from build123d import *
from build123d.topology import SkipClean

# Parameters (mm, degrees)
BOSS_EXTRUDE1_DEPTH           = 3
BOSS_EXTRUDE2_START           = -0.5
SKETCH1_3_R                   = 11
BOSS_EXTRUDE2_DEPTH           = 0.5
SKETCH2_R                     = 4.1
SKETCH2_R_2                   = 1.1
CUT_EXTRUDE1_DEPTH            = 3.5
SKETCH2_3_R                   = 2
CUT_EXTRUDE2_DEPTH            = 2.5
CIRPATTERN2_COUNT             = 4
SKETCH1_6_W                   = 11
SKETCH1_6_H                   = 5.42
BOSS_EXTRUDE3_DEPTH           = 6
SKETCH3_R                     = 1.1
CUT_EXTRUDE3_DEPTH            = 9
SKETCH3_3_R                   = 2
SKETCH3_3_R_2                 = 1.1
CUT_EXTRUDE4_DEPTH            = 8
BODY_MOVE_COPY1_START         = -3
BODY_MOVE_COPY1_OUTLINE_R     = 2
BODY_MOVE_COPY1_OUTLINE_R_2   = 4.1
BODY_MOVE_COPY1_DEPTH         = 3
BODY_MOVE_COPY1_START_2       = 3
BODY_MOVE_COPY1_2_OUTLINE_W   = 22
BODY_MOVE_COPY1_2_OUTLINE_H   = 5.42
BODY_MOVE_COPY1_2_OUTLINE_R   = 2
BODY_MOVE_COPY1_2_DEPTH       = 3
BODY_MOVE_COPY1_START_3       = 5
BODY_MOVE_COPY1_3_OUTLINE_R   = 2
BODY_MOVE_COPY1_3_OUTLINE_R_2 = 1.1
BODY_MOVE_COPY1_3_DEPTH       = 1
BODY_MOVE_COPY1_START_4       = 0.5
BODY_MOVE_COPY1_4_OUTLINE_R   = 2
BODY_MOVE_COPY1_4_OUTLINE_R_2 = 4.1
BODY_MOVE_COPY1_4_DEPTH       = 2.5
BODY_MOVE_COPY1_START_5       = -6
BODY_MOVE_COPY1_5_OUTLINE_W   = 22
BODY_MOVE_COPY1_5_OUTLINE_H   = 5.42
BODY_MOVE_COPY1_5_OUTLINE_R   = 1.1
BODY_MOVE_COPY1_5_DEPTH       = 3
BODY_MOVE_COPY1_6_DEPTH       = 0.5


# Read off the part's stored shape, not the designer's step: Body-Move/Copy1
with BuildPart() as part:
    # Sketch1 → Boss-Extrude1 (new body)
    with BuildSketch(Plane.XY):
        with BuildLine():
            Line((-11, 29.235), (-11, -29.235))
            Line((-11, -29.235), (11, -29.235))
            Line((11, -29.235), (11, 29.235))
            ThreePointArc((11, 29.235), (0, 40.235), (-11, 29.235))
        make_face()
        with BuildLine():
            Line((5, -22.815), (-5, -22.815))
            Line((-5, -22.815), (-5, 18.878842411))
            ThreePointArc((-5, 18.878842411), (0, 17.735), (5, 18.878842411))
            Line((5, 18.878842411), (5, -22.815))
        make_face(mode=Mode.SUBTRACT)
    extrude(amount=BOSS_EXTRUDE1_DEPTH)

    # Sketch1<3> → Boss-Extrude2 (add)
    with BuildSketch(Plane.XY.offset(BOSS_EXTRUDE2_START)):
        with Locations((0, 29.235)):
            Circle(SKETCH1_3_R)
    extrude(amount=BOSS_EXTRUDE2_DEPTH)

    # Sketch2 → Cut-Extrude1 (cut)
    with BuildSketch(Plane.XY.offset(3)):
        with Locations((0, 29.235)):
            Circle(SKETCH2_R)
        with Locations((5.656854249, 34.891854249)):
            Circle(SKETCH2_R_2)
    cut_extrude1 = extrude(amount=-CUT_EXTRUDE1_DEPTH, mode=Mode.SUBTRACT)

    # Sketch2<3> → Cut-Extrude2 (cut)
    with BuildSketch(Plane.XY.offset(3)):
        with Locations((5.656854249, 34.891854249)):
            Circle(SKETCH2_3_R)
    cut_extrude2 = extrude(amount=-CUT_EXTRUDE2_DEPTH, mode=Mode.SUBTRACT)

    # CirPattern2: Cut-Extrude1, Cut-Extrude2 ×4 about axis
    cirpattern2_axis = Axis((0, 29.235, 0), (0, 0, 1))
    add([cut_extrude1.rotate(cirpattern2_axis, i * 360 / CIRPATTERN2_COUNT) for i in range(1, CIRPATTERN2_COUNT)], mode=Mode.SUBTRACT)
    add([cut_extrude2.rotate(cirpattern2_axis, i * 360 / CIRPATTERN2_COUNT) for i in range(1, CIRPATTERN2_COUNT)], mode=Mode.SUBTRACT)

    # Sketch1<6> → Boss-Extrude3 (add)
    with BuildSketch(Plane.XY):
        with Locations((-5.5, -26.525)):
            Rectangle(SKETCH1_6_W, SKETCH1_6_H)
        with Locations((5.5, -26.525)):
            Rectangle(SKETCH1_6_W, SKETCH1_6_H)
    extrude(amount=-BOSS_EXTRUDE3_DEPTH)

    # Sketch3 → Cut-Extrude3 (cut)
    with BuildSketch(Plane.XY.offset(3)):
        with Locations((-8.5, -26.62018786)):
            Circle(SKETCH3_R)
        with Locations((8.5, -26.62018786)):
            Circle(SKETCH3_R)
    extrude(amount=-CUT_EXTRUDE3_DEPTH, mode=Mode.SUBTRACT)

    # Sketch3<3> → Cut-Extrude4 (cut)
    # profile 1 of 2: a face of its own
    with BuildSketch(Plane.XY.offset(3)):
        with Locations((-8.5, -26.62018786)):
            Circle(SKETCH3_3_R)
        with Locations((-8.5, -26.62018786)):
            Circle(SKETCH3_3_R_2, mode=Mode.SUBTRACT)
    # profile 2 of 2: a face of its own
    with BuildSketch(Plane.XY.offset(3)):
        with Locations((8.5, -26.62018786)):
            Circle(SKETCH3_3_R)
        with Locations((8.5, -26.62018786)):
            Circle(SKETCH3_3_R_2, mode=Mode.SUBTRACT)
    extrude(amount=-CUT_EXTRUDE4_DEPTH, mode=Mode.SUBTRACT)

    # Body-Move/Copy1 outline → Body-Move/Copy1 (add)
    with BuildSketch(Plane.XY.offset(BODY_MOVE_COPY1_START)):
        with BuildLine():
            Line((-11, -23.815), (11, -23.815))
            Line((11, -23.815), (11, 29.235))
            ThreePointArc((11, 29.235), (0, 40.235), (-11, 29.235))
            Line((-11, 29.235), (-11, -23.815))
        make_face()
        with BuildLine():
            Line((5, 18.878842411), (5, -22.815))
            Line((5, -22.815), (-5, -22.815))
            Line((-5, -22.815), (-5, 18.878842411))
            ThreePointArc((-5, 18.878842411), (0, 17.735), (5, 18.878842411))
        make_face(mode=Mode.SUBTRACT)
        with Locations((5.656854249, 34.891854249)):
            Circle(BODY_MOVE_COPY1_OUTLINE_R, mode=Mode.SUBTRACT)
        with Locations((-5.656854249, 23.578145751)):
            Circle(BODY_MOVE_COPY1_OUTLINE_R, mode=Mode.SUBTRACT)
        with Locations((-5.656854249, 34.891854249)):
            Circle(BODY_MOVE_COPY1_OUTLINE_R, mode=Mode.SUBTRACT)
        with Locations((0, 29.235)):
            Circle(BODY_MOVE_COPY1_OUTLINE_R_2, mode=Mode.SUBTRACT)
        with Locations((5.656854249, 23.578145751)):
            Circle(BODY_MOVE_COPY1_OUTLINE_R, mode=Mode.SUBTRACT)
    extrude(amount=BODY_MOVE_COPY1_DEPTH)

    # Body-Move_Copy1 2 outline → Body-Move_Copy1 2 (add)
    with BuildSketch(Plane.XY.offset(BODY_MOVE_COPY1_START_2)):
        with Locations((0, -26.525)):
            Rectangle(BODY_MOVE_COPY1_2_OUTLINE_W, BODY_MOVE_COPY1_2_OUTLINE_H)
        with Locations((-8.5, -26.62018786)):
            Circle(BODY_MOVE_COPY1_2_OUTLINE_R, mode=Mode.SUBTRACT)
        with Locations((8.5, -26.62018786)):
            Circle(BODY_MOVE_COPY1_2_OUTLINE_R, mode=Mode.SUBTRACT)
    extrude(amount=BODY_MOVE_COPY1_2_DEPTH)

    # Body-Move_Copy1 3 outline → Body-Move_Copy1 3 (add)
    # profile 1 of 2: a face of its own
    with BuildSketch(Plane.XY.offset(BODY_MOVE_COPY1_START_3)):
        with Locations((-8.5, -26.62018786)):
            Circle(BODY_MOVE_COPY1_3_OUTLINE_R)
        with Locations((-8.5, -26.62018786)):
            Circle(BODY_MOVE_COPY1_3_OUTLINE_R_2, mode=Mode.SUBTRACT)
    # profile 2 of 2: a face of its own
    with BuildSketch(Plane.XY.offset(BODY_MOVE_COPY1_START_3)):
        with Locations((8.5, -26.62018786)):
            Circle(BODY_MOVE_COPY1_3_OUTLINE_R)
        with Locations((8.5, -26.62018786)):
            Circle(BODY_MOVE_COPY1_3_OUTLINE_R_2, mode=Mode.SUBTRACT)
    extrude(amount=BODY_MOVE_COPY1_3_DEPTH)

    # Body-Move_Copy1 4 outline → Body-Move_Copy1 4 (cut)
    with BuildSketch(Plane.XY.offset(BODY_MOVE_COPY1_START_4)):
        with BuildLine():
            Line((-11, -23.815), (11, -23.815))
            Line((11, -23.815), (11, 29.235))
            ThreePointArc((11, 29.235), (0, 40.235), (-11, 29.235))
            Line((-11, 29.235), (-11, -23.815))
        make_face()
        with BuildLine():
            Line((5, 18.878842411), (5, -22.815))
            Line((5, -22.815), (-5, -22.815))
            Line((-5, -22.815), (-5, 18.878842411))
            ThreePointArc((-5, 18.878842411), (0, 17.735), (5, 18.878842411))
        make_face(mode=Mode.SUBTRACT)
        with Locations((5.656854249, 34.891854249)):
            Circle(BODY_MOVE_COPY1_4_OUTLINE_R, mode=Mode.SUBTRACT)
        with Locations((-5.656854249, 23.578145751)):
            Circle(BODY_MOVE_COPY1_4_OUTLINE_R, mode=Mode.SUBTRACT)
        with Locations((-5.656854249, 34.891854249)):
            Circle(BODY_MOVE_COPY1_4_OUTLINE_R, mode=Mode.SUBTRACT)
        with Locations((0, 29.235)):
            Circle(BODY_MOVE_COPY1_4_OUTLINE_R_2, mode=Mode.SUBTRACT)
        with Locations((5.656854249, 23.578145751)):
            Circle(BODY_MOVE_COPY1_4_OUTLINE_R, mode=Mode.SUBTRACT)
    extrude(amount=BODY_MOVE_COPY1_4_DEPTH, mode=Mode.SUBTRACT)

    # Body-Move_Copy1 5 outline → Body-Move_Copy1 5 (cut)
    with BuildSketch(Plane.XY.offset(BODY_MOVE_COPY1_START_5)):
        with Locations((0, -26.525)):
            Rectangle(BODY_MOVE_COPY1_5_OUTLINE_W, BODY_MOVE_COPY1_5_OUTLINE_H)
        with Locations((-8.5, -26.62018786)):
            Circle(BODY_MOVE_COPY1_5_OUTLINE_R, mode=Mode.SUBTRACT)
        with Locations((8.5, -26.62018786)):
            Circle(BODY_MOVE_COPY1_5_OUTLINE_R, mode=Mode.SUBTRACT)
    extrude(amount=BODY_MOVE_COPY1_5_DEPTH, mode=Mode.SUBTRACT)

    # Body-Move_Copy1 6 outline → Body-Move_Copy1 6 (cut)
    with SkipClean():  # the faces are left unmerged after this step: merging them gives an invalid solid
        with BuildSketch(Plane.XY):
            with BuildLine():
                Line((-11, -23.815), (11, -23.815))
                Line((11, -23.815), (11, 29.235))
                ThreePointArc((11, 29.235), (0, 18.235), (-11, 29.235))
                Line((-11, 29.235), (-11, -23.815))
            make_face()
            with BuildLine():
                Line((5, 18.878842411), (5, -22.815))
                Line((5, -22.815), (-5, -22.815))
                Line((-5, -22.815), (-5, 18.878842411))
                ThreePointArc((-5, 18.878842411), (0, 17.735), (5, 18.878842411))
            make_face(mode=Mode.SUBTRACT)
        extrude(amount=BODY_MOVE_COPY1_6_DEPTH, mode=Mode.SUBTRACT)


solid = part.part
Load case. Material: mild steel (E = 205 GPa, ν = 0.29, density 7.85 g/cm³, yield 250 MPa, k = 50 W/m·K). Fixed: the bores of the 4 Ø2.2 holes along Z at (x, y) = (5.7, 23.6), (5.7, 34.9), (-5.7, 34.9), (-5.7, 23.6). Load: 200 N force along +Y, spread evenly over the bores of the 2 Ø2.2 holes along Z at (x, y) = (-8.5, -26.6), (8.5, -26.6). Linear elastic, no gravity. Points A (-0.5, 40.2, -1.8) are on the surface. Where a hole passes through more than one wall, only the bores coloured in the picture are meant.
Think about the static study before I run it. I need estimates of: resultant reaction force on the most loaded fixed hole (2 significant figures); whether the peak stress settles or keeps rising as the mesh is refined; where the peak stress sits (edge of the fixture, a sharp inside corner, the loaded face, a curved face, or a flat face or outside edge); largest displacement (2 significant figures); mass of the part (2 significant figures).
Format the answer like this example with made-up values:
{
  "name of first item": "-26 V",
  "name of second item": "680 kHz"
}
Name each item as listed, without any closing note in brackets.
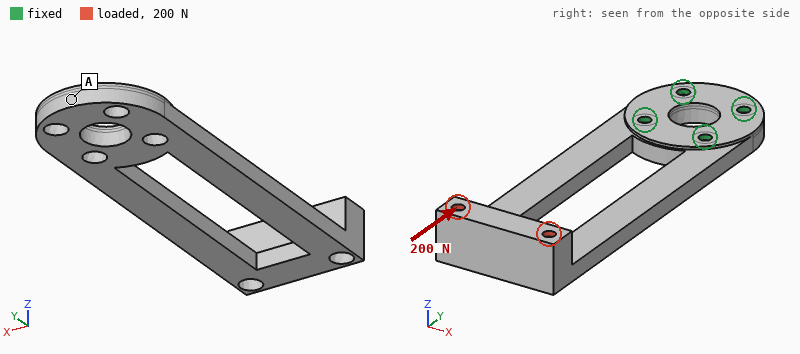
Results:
{
  "resultant reaction force on the most loaded fixed hole": "160 N",
  "whether the peak stress settles or keeps rising as the mesh is refined": "keeps rising",
  "where the peak stress sits": "edge of the fixture",
  "largest displacement": "0.36 mm",
  "mass of the part": "28 g"
}
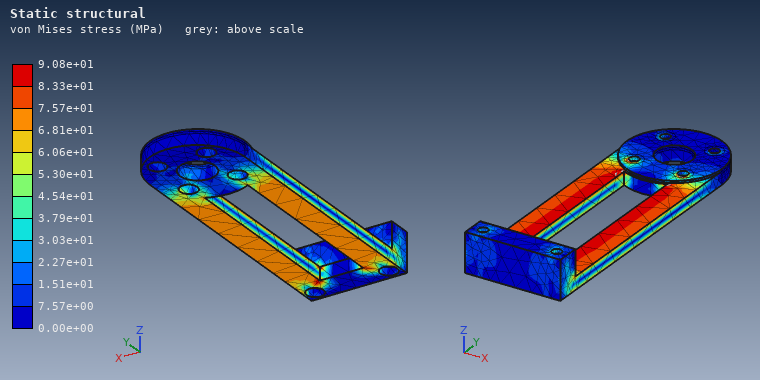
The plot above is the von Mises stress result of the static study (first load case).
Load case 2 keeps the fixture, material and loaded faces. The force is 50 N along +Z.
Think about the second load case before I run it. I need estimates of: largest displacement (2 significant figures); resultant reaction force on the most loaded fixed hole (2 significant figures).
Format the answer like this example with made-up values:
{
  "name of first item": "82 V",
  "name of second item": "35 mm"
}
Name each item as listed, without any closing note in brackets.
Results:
{
  "largest displacement": "0.42 mm",
  "resultant reaction force on the most loaded fixed hole": "200 N"
}
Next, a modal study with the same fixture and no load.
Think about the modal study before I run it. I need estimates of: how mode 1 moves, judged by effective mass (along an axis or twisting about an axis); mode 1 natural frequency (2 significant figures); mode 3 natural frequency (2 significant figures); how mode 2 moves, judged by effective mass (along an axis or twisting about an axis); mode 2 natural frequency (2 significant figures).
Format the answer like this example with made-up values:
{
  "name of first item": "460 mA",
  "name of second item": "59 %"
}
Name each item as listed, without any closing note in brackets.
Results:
{
  "how mode 1 moves, judged by effective mass": "along Z",
  "mode 1 natural frequency": "580 Hz",
  "mode 3 natural frequency": "2600 Hz",
  "how mode 2 moves, judged by effective mass": "along X",
  "mode 2 natural frequency": "1900 Hz"
}
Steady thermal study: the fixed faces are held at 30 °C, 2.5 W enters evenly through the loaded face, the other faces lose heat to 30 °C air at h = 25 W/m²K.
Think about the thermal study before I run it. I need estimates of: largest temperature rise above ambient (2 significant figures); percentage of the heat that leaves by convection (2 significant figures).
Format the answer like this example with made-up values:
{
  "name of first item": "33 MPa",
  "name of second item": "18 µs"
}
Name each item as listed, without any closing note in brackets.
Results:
{
  "largest temperature rise above ambient": "44 K",
  "percentage of the heat that leaves by convection": "60 %"
}
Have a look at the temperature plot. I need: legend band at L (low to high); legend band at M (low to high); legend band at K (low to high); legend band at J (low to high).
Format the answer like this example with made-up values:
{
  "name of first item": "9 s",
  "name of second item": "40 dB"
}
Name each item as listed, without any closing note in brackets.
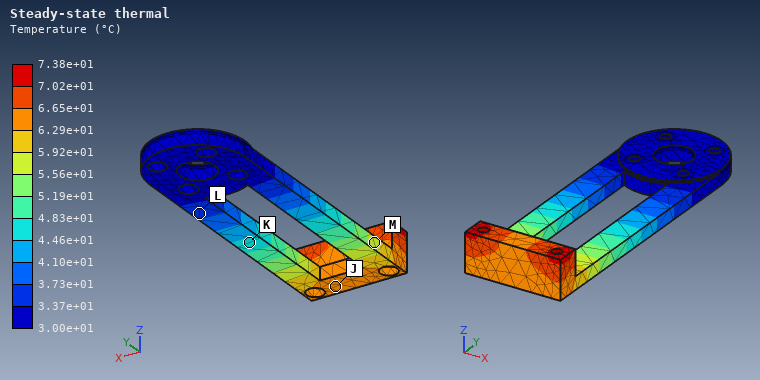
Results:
{
  "legend band at L": "3.37e+01 to 3.73e+01 °C",
  "legend band at M": "5.56e+01 to 5.92e+01 °C",
  "legend band at K": "4.46e+01 to 4.83e+01 °C",
  "legend band at J": "6.29e+01 to 6.65e+01 °C"
}
